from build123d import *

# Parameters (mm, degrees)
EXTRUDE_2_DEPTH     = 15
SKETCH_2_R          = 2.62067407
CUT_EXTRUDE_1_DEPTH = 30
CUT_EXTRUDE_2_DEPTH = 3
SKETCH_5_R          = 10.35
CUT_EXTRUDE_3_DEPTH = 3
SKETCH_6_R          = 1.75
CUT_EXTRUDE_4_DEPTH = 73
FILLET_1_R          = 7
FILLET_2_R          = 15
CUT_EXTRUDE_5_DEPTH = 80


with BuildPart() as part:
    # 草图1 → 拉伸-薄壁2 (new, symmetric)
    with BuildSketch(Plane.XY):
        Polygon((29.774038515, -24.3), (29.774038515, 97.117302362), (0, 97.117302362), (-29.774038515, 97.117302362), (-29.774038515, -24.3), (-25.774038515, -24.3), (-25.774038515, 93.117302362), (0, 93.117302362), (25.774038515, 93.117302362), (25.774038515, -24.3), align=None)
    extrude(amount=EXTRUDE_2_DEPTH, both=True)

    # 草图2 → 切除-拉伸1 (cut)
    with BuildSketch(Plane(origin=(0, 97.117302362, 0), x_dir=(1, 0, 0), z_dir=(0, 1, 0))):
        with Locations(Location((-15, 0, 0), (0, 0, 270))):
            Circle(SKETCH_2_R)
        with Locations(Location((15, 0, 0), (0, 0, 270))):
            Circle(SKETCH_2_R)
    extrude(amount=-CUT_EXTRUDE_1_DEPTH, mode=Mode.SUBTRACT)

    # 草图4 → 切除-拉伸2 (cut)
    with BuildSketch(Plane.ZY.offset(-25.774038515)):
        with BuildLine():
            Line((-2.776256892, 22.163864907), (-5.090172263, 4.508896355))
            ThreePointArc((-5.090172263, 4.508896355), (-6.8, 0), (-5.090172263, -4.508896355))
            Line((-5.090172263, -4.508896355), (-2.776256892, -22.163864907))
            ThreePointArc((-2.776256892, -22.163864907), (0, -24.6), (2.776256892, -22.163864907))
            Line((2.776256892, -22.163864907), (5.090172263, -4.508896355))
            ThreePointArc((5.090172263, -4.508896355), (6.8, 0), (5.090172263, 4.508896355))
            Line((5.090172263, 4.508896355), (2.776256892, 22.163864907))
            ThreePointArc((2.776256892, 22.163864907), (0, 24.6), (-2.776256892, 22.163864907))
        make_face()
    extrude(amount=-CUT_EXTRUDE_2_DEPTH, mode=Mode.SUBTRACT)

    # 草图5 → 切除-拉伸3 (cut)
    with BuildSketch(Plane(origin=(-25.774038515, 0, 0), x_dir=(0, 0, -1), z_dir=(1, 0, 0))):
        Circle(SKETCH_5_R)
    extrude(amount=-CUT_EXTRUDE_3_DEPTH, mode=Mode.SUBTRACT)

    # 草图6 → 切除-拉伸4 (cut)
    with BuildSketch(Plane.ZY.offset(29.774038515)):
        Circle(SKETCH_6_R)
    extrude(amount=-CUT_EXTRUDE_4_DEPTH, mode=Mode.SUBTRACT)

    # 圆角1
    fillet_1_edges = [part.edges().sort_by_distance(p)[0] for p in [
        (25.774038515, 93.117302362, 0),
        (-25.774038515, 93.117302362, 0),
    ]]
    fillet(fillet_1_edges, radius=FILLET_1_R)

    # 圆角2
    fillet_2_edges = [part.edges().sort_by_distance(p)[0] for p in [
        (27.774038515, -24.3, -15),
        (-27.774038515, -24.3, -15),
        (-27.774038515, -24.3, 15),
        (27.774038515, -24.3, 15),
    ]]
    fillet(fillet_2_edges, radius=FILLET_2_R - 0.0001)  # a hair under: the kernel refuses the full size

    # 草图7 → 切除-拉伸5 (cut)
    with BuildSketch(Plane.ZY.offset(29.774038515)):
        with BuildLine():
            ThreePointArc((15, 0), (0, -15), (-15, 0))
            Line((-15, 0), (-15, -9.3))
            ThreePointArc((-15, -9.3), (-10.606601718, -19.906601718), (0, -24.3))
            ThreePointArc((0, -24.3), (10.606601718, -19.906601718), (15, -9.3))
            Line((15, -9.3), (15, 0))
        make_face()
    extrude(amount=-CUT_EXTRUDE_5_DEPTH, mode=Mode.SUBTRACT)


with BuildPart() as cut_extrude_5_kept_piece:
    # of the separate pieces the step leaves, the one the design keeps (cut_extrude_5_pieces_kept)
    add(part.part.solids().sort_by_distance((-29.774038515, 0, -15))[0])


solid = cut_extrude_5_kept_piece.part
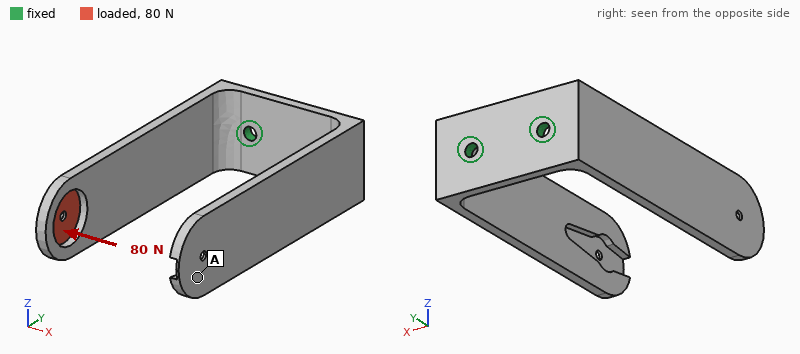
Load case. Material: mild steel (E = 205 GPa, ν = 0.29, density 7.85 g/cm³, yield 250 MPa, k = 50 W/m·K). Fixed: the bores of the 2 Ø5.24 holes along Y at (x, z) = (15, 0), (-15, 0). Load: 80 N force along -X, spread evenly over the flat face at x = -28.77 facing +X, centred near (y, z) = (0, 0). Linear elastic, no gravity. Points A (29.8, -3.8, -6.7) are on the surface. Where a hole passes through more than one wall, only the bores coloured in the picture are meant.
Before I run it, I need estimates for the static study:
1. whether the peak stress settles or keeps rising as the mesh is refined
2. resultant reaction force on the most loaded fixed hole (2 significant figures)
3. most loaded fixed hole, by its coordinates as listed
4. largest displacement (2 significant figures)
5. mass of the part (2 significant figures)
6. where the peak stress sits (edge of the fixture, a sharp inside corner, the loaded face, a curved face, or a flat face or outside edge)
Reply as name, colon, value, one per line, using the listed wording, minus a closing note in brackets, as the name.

whether the peak stress settles or keeps rising as the mesh is refined: keeps rising
resultant reaction force on the most loaded fixed hole: 110 N
most loaded fixed hole, by its coordinates as listed: (-15, 0)
largest displacement: 0.96 mm
mass of the part: 240 g
where the peak stress sits: edge of the fixture
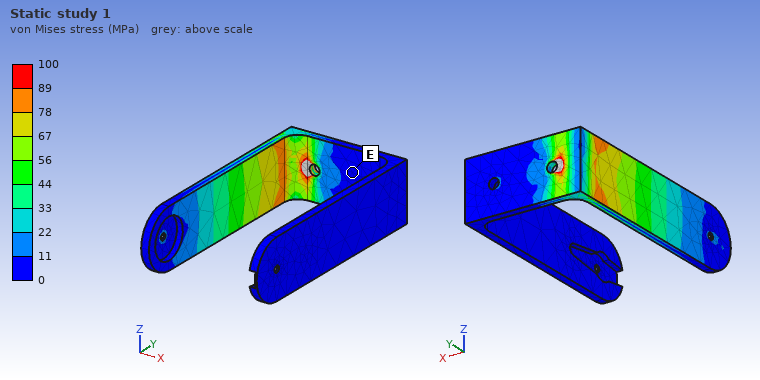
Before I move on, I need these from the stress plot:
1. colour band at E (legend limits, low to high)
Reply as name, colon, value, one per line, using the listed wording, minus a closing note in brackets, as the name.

colour band at E: 0 to 11 MPa
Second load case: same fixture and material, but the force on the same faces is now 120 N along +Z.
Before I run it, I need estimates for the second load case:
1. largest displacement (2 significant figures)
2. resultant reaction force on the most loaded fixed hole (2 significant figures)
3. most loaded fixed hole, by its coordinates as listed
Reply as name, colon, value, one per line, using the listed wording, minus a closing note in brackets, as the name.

largest displacement: 0.21 mm
resultant reaction force on the most loaded fixed hole: 150 N
most loaded fixed hole, by its coordinates as listed: (-15, 0)
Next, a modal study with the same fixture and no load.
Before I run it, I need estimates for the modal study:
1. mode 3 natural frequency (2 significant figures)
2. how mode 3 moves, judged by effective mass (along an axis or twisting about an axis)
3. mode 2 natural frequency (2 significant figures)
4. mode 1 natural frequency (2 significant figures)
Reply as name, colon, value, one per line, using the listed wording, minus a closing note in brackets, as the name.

mode 3 natural frequency: 700 Hz
how mode 3 moves, judged by effective mass: along Z
mode 2 natural frequency: 310 Hz
mode 1 natural frequency: 310 Hz
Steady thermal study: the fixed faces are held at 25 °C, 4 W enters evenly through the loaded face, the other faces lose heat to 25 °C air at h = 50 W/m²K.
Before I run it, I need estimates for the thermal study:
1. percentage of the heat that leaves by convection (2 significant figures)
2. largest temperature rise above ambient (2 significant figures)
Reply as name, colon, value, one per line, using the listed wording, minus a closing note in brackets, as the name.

percentage of the heat that leaves by convection: 88 %
largest temperature rise above ambient: 28 K
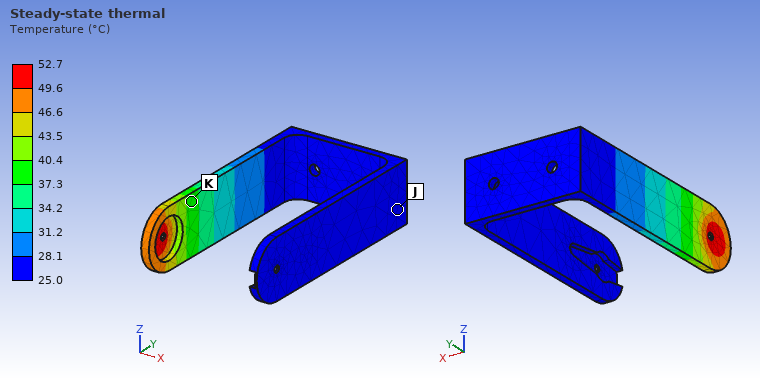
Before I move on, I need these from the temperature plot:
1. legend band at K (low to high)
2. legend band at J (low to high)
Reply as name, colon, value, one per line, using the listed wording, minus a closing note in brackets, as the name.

legend band at K: 37.3 to 40.4 °C
legend band at J: 25.0 to 28.1 °C
